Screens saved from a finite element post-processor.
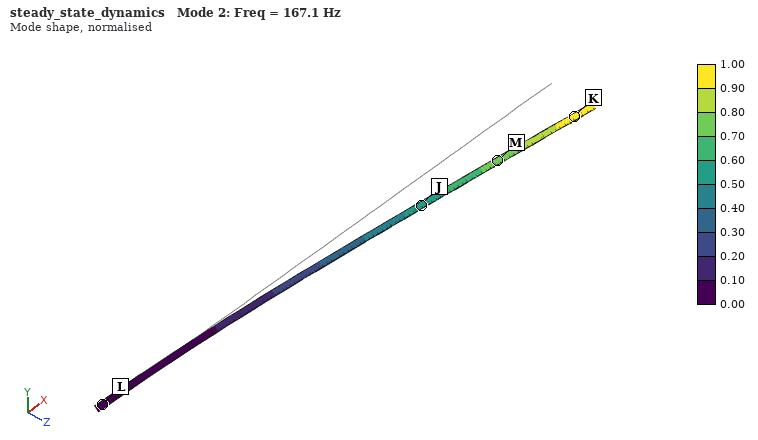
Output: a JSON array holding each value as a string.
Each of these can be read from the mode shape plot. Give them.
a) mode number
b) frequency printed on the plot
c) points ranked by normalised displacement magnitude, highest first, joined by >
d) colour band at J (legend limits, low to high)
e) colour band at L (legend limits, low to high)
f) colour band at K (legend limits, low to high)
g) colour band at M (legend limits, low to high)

["2", "167.1 Hz", "K > M > J > L", "0.50 to 0.60", "0.00 to 0.10", "0.90 to 1.00", "0.70 to 0.80"]
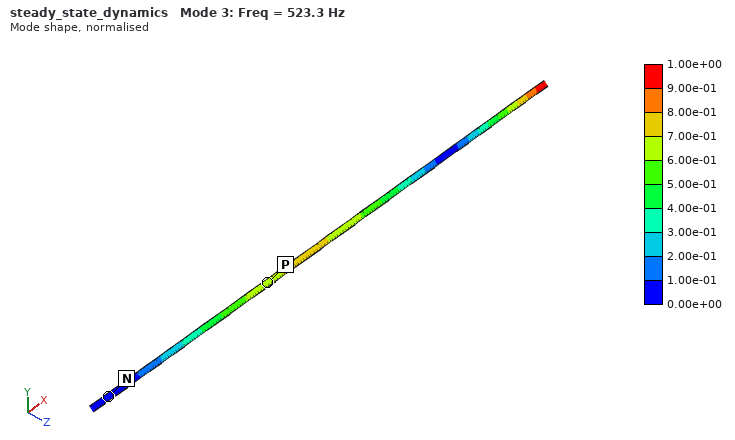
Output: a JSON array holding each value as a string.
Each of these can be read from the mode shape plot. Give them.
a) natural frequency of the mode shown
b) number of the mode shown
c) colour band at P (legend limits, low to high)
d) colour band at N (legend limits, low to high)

["523.3 Hz", "3", "6.00e-01 to 7.00e-01", "0.00e+00 to 1.00e-01"]
